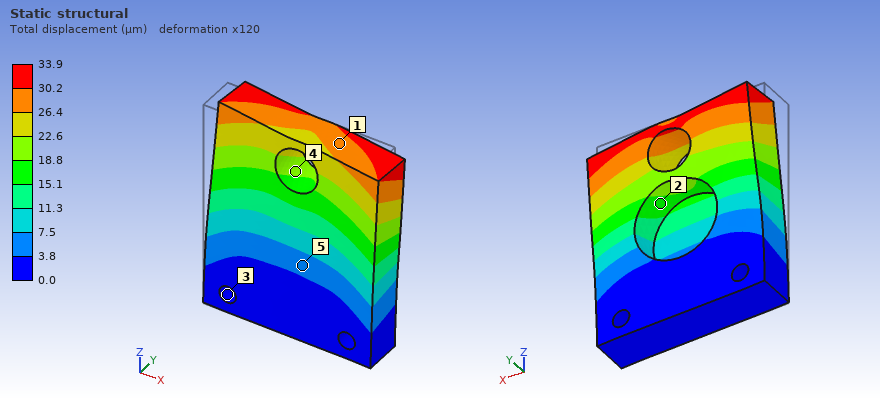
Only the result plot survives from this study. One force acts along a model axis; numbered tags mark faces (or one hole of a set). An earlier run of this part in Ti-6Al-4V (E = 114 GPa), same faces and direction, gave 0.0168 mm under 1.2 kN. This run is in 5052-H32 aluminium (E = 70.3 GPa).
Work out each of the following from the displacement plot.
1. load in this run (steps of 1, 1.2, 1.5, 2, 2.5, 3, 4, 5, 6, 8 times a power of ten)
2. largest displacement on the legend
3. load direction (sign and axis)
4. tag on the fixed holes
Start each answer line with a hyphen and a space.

- 1.5 kN
- 33.9 µm
- +X
- 3
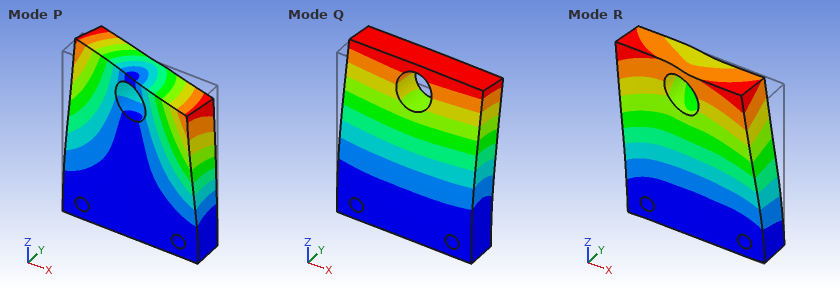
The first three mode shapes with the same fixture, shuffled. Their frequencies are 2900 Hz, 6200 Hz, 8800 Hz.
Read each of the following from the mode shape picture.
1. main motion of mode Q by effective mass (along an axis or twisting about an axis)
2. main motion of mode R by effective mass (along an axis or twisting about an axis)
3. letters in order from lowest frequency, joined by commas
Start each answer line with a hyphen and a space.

- along Y
- along X
- Q, P, R
